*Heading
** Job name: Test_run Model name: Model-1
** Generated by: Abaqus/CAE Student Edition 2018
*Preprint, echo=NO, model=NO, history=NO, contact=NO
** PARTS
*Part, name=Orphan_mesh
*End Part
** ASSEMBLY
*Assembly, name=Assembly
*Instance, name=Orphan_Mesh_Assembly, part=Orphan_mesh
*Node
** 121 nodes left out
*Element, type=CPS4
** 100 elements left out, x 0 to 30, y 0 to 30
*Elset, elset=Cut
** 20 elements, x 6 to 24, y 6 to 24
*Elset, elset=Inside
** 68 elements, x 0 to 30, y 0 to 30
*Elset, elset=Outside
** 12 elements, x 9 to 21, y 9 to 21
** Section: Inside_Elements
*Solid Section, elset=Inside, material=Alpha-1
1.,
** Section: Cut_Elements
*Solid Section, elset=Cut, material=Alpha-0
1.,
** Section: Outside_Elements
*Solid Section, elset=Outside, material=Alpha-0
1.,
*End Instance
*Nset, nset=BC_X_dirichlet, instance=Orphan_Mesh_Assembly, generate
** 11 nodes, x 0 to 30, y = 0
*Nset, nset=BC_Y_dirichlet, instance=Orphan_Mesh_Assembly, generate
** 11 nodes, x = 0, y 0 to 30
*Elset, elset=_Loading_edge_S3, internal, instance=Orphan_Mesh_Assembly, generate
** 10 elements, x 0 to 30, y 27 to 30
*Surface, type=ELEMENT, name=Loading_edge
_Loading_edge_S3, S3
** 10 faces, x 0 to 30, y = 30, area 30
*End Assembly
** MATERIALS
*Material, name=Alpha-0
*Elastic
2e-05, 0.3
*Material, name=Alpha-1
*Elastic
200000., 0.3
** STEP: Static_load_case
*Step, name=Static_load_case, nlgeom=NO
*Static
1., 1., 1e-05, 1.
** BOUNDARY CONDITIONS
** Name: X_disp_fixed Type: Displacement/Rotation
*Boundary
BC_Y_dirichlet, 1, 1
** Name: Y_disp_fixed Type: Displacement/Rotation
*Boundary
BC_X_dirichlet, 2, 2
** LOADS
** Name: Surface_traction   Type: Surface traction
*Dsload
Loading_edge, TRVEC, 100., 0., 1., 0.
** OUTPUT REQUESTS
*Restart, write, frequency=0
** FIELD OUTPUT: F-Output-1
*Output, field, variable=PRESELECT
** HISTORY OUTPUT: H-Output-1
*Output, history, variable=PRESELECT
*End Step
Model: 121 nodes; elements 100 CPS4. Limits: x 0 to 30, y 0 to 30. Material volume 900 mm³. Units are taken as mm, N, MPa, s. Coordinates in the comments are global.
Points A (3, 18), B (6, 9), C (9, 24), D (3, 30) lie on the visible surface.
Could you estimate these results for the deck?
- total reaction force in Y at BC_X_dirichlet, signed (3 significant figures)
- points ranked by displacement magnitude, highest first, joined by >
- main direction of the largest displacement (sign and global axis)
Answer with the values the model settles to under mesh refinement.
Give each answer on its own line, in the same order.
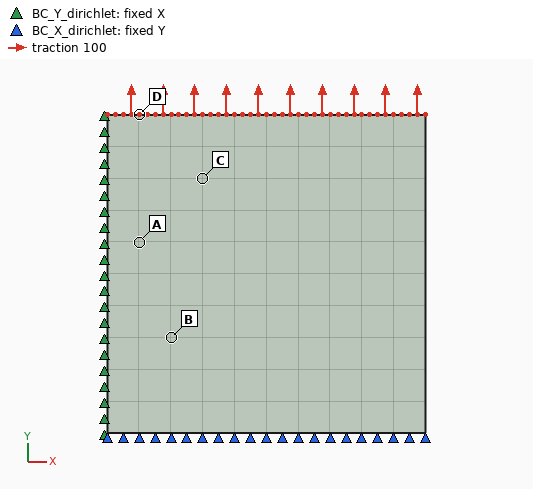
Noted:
-3000 N
C > D > A > B
+Y
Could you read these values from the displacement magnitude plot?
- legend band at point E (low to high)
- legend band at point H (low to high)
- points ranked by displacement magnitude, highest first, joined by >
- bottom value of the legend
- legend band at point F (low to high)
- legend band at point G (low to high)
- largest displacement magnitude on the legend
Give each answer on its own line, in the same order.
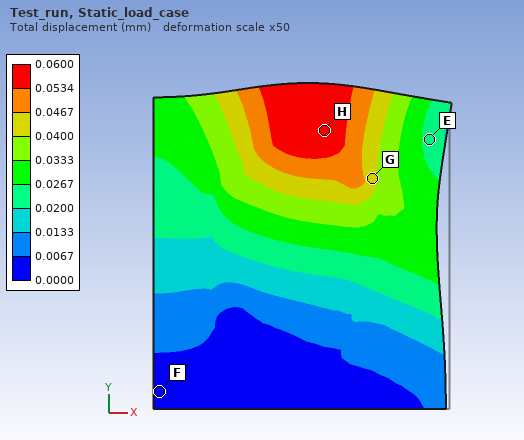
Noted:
0.0200 to 0.0267 mm
0.0534 to 0.0600 mm
H > G > E > F
0.0000 mm
0.0000 to 0.0067 mm
0.0400 to 0.0467 mm
0.0600 mm
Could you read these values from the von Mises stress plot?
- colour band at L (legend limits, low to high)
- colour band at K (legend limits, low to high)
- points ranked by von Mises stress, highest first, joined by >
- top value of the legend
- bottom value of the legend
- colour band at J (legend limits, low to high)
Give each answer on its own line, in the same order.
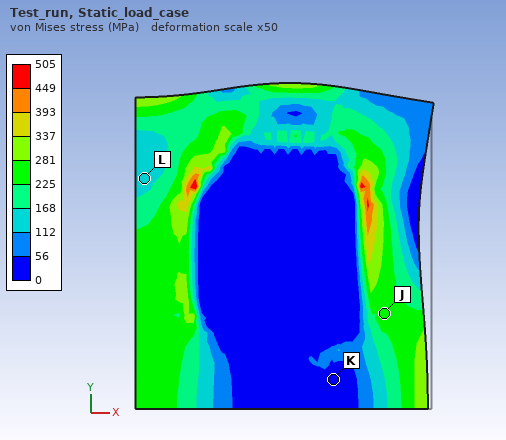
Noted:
112 to 168 MPa
0 to 56 MPa
J > L > K
505 MPa
0 MPa
225 to 281 MPa
